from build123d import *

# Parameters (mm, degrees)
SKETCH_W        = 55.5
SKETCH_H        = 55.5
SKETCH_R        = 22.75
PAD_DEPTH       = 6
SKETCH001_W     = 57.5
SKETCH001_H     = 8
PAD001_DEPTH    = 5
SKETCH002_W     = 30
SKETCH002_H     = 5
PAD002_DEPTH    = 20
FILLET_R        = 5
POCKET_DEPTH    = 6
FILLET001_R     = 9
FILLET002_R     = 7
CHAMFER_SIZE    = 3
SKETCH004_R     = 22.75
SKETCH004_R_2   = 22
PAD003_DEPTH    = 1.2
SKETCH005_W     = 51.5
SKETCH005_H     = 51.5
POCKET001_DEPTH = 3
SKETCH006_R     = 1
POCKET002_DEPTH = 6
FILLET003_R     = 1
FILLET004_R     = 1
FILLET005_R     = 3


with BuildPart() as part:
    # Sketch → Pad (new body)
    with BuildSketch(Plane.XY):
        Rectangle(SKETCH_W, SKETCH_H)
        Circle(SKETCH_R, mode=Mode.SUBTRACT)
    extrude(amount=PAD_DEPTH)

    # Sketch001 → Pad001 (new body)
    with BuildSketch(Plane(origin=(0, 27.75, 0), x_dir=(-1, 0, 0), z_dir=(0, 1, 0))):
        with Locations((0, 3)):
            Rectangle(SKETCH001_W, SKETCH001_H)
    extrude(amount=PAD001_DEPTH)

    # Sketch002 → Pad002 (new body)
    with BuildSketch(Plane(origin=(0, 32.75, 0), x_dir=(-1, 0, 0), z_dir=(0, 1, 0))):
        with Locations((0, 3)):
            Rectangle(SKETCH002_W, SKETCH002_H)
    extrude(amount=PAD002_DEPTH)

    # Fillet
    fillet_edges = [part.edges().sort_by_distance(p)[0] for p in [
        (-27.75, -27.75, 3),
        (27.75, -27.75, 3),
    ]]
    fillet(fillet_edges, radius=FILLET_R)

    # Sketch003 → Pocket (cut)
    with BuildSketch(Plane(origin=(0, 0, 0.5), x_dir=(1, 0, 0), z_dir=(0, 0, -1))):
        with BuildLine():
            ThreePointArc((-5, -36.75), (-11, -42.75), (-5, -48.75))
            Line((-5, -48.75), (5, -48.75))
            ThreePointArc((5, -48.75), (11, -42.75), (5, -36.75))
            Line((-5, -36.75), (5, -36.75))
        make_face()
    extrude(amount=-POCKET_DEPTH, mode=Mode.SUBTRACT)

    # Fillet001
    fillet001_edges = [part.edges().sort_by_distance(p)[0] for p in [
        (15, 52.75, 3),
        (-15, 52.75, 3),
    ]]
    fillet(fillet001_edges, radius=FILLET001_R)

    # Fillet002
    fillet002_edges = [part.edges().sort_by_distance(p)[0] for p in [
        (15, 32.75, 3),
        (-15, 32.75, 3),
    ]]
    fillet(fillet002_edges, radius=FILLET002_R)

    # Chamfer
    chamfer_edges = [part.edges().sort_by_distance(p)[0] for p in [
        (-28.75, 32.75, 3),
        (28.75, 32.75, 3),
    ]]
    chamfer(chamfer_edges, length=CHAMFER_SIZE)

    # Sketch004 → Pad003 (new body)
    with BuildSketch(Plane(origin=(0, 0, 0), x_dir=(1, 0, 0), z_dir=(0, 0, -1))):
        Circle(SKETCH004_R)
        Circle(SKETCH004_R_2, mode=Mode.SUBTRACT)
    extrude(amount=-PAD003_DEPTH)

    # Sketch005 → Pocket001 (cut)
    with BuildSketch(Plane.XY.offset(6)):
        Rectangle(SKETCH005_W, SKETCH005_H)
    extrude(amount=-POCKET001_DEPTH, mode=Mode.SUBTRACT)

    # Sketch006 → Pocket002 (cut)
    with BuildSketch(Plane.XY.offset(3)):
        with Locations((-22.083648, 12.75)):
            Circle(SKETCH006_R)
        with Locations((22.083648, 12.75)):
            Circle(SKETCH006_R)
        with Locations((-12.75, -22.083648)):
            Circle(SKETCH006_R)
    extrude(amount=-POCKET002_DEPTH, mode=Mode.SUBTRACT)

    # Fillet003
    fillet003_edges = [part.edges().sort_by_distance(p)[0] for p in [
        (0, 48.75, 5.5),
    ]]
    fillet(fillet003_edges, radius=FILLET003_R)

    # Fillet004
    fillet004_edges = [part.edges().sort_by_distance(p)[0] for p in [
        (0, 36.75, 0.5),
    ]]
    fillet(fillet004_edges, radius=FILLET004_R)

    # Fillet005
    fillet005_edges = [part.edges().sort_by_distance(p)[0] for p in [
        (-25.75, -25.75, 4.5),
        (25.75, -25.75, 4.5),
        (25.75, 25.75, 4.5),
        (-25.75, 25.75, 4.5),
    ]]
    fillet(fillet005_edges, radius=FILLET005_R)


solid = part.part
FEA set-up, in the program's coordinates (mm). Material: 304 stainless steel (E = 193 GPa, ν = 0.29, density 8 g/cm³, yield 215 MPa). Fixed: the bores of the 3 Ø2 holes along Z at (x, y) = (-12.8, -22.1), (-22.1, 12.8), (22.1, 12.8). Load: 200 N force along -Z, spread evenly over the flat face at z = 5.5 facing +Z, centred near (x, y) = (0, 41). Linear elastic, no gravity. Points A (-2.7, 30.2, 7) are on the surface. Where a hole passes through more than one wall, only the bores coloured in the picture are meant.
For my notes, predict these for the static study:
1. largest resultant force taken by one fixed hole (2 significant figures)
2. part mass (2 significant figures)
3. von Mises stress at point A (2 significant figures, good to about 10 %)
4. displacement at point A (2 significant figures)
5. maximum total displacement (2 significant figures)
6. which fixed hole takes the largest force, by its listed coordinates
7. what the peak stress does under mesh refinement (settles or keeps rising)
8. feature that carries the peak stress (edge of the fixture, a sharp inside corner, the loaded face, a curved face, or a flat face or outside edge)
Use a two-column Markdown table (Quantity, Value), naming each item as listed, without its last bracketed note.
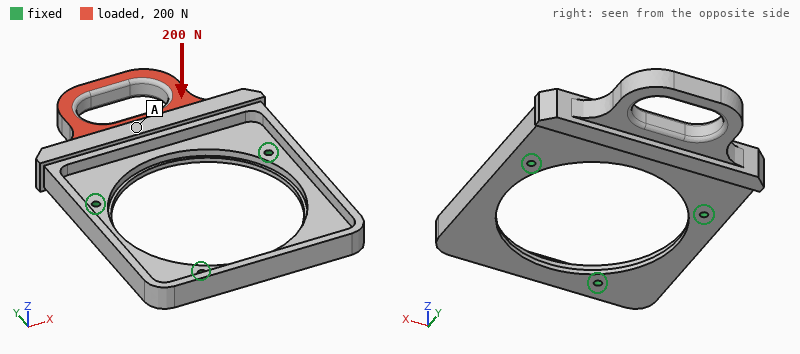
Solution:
| Quantity | Value |
|---|---|
| largest resultant force taken by one fixed hole | 150 N |
| part mass | 77 g |
| von Mises stress at point A | 14 MPa |
| displacement at point A | 0.047 mm |
| maximum total displacement | 0.13 mm |
| which fixed hole takes the largest force, by its listed coordinates | (-22.1, 12.8) |
| what the peak stress does under mesh refinement | keeps rising |
| feature that carries the peak stress | edge of the fixture |
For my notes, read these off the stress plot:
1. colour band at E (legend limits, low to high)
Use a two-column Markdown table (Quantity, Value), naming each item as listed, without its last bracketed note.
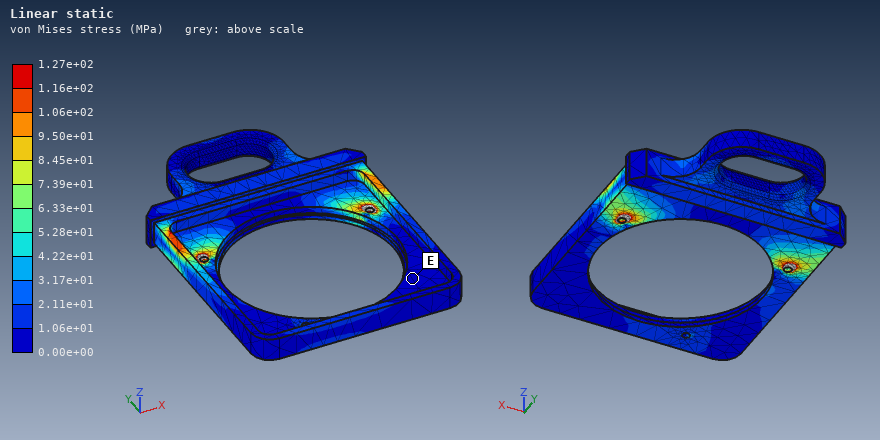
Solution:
| Quantity | Value |
|---|---|
| colour band at E | 0.00e+00 to 1.06e+01 MPa |
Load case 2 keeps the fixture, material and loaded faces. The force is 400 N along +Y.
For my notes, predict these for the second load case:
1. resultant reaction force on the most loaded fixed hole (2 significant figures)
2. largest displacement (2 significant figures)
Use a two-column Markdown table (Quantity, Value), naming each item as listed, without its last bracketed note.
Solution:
| Quantity | Value |
|---|---|
| resultant reaction force on the most loaded fixed hole | 220 N |
| largest displacement | 44 µm |
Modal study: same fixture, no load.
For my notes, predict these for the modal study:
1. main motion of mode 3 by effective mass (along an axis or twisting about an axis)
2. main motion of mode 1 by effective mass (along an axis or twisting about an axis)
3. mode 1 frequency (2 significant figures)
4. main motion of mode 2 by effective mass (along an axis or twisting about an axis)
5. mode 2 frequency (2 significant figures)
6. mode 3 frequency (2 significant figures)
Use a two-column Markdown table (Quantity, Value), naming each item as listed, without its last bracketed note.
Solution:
| Quantity | Value |
|---|---|
| main motion of mode 3 by effective mass | twisting about Y |
| main motion of mode 1 by effective mass | along Z |
| mode 1 frequency | 1700 Hz |
| main motion of mode 2 by effective mass | along Z |
| mode 2 frequency | 2500 Hz |
| mode 3 frequency | 6000 Hz |
